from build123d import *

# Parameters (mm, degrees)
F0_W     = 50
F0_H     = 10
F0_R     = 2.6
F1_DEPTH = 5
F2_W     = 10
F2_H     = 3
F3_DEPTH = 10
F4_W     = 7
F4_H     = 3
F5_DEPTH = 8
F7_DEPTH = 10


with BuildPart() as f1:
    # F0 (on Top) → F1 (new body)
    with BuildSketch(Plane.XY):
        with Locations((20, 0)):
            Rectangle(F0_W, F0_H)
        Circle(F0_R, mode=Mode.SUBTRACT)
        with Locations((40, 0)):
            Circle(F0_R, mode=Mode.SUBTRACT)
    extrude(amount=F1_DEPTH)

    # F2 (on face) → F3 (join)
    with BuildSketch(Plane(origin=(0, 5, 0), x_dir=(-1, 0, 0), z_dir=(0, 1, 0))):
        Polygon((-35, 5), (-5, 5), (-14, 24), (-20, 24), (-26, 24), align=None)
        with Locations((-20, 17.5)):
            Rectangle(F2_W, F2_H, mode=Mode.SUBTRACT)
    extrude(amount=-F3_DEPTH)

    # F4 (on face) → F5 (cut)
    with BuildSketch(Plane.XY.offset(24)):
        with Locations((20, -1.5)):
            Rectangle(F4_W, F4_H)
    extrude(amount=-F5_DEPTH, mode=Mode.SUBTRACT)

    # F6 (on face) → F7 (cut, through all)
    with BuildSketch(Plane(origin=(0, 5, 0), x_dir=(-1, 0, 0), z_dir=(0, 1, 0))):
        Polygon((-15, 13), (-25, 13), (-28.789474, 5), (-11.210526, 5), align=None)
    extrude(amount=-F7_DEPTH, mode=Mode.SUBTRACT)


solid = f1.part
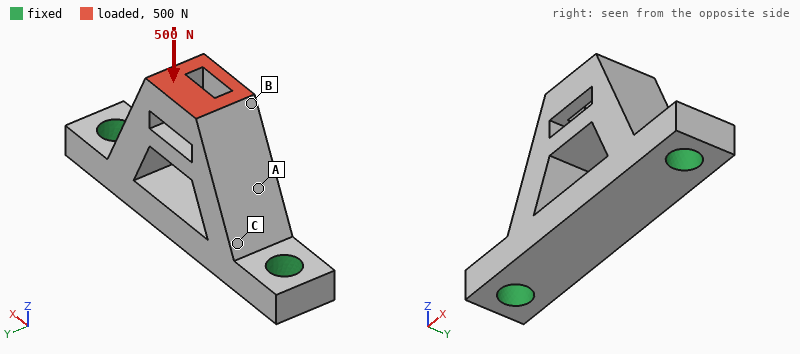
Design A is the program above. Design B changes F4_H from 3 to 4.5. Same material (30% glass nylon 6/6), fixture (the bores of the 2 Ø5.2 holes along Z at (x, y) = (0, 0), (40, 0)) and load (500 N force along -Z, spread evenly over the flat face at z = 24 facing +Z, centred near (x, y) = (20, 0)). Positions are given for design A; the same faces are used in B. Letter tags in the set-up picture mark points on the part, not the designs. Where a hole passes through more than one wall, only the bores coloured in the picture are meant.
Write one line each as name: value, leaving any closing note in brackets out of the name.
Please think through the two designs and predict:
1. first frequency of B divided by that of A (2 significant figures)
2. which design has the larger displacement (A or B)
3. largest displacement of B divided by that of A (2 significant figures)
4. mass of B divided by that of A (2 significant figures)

first frequency of B divided by that of A: 1.0
which design has the larger displacement: B
largest displacement of B divided by that of A: 1.2
mass of B divided by that of A: 0.99
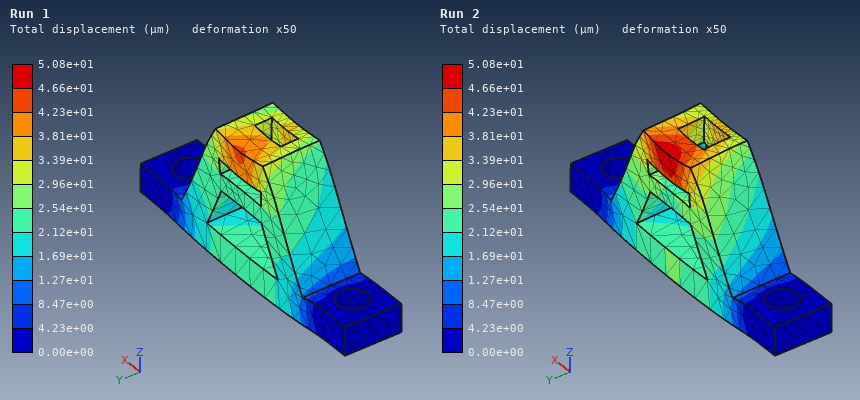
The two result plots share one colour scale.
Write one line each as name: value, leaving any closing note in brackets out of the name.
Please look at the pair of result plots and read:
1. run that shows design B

run that shows design B: Run 2
